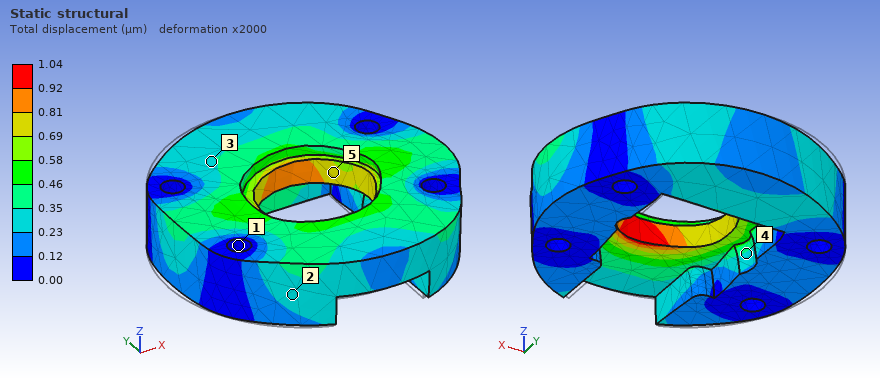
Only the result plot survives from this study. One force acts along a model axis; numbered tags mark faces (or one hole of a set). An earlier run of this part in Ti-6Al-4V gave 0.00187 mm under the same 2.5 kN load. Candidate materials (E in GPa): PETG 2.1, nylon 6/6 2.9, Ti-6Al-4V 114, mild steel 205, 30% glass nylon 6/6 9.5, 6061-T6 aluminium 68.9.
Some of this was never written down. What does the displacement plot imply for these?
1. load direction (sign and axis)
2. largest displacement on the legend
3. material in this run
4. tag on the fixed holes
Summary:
+X
1.04 µm
mild steel
1
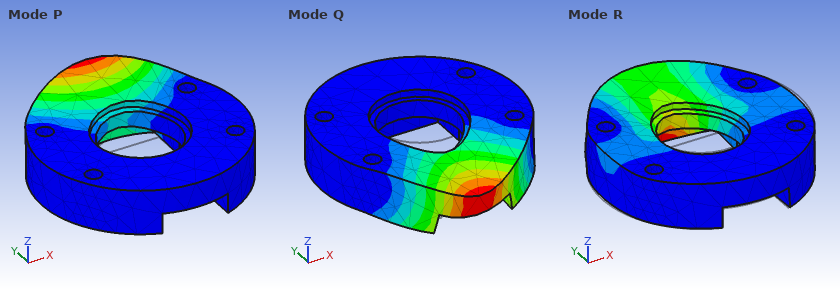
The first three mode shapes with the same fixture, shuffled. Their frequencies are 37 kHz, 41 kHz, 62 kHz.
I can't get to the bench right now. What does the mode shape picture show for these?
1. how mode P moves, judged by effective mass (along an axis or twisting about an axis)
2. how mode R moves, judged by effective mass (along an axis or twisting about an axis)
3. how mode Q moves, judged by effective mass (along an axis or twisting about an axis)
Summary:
along Z
along Y
along Z
